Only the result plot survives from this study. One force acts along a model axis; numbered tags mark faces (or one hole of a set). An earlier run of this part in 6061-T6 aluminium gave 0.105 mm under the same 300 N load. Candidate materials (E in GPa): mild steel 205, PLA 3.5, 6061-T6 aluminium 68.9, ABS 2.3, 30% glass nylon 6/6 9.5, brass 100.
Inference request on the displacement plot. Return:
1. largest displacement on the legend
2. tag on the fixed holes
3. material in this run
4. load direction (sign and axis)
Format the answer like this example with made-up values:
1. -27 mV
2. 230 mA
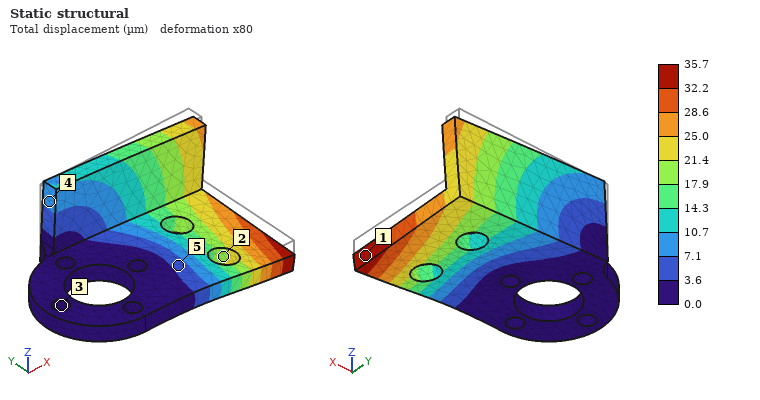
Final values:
1. 35.7 µm
2. 3
3. mild steel
4. -Z
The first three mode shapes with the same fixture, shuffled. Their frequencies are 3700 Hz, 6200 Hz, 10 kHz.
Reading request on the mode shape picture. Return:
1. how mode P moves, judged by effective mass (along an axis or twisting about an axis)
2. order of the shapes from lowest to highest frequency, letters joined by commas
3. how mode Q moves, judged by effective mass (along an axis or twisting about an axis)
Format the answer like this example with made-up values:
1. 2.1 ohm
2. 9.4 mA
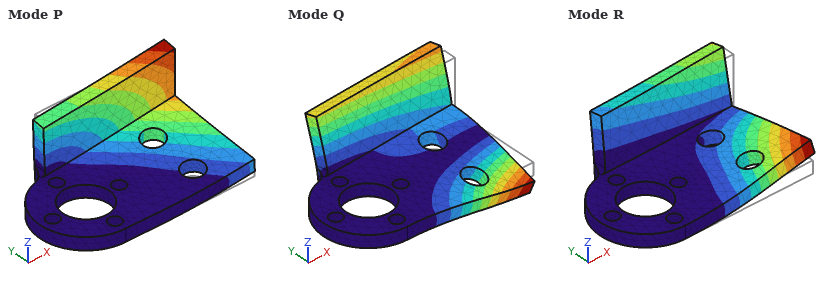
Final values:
1. along Z
2. P, R, Q
3. along Y
